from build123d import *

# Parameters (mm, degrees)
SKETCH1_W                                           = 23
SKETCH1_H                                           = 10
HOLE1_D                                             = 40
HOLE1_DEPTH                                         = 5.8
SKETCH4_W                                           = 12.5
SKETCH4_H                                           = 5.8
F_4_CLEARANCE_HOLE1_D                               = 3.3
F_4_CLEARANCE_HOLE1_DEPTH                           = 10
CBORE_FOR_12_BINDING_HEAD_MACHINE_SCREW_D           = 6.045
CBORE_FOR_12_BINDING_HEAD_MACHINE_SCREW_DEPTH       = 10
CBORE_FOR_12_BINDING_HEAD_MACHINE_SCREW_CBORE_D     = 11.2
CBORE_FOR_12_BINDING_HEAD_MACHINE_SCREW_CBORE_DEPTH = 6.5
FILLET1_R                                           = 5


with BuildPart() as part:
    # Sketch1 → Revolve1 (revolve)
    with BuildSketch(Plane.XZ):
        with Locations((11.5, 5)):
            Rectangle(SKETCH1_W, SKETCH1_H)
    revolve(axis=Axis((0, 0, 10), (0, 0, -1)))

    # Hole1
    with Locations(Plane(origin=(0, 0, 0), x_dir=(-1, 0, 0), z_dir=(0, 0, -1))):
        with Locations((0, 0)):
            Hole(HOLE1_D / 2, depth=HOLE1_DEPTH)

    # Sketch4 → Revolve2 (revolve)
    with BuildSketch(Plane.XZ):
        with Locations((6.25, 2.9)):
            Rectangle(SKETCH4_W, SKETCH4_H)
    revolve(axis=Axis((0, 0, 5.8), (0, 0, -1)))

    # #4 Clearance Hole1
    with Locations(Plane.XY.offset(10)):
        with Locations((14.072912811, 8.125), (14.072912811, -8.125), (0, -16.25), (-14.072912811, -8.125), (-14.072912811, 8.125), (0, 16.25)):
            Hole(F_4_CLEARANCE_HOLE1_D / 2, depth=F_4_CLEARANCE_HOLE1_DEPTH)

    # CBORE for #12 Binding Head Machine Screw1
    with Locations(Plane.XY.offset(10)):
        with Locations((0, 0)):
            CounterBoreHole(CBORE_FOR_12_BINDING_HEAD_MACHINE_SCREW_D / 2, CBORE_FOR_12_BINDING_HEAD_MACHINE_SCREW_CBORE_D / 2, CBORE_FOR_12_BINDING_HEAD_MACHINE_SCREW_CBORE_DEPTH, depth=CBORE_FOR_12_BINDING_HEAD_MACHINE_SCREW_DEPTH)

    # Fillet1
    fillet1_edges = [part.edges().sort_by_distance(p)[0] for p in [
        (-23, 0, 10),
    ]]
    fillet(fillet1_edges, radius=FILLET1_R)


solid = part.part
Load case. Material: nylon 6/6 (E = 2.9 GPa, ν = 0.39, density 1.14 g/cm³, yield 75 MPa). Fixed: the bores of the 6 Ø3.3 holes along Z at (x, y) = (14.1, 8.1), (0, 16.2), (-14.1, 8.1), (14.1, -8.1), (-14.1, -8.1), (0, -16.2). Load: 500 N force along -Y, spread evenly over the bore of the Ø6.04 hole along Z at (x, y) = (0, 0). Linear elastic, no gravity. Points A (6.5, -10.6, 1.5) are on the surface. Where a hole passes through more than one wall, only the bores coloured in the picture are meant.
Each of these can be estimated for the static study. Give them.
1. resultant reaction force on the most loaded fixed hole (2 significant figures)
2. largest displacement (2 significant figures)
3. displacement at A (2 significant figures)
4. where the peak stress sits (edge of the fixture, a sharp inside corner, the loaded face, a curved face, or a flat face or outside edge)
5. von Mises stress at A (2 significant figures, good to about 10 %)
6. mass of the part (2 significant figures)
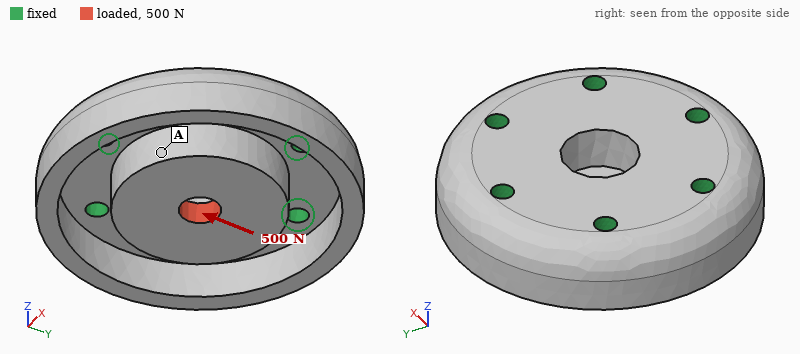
140 N
35 µm
18 µm
a sharp inside corner
1.7 MPa
12 g
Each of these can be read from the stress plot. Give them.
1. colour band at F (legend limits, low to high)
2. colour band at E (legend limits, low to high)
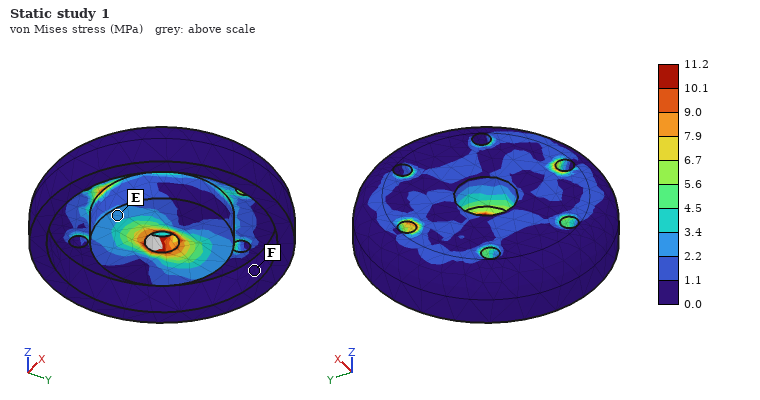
0.0 to 1.1 MPa
2.2 to 3.4 MPa
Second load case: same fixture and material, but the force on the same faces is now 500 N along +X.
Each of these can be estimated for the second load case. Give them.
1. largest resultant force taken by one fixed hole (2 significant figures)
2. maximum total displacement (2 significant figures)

120 N
35 µm
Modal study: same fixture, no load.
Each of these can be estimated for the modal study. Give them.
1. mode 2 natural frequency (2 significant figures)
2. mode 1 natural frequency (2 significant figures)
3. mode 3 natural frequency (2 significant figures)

8700 Hz
8700 Hz
8800 Hz
